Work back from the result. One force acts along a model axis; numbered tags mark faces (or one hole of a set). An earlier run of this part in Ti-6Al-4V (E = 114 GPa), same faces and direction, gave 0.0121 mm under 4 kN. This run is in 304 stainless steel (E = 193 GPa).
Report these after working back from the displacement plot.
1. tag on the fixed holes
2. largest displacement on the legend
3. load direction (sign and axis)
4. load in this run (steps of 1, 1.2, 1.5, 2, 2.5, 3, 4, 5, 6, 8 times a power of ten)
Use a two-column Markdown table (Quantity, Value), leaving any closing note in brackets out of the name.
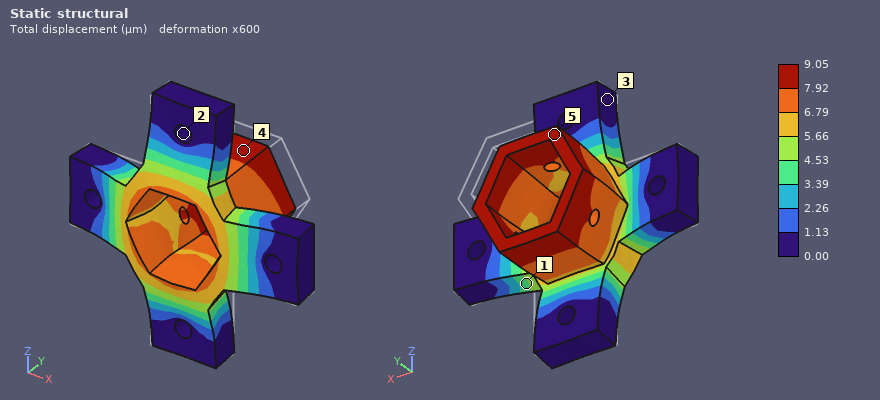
| Quantity | Value |
|---|---|
| tag on the fixed holes | 2 |
| largest displacement on the legend | 9.05 µm |
| load direction | -Y |
| load in this run | 5 kN |
